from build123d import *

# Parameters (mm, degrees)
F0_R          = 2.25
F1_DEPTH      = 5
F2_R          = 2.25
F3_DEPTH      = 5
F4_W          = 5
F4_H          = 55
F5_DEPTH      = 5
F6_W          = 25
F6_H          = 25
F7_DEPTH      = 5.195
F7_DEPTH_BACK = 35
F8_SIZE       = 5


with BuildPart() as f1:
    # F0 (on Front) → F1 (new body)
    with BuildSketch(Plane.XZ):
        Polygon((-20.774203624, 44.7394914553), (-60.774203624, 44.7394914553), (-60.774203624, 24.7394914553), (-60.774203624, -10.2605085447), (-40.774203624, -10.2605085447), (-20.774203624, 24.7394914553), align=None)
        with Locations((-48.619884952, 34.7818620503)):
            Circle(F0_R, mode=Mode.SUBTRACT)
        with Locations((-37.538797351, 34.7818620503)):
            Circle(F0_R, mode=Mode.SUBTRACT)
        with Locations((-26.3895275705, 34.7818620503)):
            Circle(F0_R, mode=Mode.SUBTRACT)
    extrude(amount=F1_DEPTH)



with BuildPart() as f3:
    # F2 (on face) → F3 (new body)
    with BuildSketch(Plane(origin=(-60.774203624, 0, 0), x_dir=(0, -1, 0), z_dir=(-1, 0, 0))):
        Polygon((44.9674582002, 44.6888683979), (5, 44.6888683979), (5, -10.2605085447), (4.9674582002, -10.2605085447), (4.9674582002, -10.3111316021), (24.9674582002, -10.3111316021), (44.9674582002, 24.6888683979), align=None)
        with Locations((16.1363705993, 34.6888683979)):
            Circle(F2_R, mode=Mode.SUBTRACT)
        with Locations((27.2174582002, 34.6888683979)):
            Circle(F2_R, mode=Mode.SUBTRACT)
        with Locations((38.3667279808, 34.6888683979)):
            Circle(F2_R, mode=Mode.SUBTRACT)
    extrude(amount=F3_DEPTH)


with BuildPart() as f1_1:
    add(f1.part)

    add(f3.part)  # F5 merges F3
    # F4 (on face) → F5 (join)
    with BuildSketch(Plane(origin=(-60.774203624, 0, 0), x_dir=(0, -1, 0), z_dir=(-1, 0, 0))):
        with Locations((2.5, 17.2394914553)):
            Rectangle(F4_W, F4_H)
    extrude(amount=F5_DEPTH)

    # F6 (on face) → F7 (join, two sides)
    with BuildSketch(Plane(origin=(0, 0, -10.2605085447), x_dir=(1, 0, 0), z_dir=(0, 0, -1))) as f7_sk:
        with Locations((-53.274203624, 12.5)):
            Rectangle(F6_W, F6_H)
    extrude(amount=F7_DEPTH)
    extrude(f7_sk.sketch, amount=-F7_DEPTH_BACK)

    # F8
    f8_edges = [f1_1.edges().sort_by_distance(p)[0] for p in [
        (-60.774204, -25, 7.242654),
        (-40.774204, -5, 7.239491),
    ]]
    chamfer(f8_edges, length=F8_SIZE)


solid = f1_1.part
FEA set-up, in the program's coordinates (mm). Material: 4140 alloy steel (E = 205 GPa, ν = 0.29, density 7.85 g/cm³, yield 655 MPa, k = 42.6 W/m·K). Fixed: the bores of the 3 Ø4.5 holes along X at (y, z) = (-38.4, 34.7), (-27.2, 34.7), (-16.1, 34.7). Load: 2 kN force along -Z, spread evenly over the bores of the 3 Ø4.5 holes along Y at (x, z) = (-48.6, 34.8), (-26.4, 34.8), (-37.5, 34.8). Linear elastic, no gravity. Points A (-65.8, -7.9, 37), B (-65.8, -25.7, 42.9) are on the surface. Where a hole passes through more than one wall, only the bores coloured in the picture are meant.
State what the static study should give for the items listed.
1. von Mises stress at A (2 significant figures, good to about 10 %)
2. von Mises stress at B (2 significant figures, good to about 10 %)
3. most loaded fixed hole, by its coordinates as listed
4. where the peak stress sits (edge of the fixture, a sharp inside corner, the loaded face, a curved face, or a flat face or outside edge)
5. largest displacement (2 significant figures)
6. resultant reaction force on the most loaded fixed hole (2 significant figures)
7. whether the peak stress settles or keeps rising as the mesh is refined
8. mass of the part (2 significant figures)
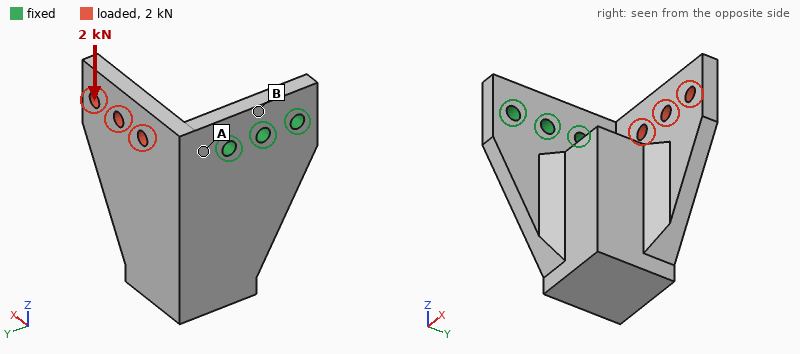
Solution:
170 MPa
49 MPa
(-16.1, 34.7)
edge of the fixture
0.27 mm
2.7 kN
keeps rising
290 g
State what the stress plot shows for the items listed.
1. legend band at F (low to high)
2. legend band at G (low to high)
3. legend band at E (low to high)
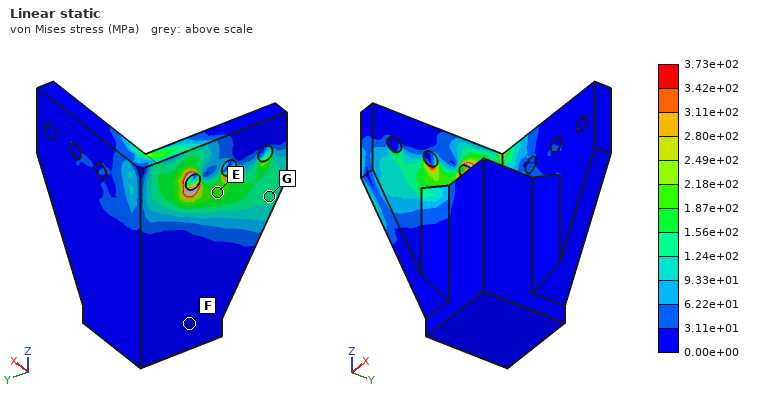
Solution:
0.00e+00 to 3.11e+01 MPa
1.24e+02 to 1.56e+02 MPa
1.87e+02 to 2.18e+02 MPa
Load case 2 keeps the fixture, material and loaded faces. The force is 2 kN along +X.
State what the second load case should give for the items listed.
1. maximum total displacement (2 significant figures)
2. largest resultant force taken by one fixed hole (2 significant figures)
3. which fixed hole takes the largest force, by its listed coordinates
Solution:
53 µm
2.8 kN
(-16.1, 34.7)
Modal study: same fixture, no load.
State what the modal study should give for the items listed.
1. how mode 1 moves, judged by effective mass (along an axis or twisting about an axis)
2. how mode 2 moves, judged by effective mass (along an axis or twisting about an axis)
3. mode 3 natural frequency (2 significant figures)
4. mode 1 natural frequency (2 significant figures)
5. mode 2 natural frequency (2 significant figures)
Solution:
along X
along Y
4900 Hz
1000 Hz
2800 Hz
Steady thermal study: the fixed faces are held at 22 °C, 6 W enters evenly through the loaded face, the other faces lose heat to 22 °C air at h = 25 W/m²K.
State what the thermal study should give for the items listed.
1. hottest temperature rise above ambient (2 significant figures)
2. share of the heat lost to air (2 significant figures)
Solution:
22 K
32 %
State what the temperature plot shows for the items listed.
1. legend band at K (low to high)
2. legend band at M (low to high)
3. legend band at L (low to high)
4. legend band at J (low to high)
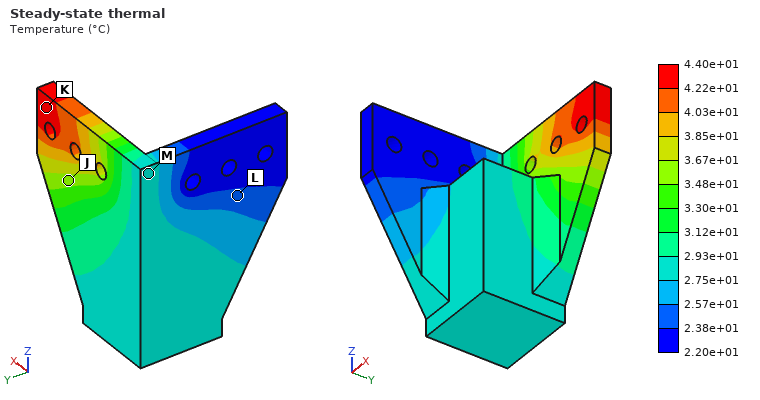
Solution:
4.22e+01 to 4.40e+01 °C
2.75e+01 to 2.93e+01 °C
2.38e+01 to 2.57e+01 °C
3.48e+01 to 3.67e+01 °C
